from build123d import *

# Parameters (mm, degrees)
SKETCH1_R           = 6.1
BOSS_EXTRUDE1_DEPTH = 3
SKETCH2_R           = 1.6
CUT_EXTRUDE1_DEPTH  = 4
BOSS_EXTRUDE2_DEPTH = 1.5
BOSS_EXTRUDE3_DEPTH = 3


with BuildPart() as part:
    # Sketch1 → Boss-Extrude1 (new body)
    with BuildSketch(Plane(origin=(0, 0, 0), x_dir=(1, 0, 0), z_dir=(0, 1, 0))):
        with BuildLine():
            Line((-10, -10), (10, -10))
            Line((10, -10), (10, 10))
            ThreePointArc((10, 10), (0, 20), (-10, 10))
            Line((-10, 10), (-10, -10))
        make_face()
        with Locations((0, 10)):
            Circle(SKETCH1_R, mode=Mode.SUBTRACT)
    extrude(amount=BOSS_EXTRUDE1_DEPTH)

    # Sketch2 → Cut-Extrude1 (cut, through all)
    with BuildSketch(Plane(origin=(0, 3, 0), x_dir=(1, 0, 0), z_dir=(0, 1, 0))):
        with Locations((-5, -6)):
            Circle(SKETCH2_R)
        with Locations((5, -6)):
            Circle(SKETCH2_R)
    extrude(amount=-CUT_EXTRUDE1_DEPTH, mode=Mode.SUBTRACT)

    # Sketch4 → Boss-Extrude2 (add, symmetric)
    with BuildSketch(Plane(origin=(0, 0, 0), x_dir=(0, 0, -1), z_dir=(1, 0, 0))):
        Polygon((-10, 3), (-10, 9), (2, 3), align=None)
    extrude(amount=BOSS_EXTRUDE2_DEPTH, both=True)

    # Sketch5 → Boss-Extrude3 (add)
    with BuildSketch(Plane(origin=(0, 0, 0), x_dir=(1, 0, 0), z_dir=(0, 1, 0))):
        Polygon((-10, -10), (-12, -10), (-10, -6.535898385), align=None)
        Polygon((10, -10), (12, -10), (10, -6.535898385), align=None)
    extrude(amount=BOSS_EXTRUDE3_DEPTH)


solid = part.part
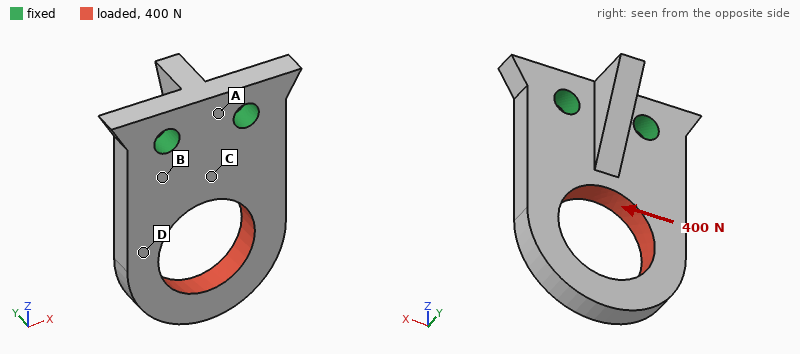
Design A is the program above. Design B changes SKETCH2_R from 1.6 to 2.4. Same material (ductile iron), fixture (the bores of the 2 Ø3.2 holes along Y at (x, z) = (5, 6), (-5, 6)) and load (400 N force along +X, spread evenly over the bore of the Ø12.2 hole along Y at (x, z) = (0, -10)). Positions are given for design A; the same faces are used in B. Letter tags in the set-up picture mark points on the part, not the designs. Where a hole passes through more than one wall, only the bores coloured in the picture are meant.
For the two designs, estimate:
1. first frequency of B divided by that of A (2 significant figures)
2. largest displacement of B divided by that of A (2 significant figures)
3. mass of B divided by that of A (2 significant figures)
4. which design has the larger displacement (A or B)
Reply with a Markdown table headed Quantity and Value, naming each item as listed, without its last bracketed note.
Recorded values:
| Quantity | Value |
|---|---|
| first frequency of B divided by that of A | 1.1 |
| largest displacement of B divided by that of A | 0.91 |
| mass of B divided by that of A | 0.96 |
| which design has the larger displacement | A |
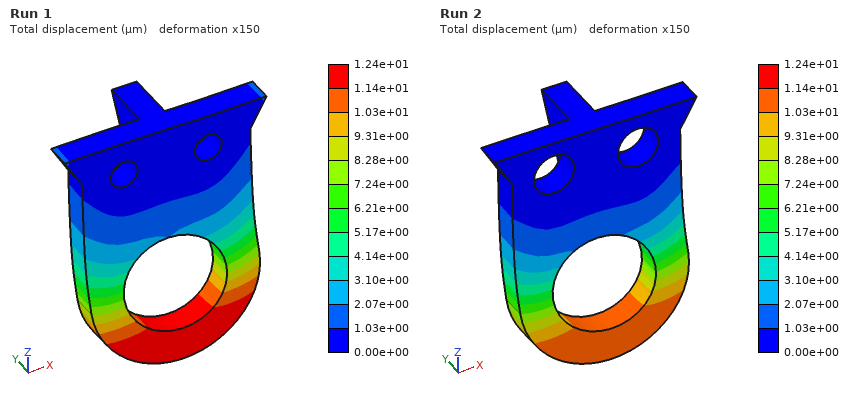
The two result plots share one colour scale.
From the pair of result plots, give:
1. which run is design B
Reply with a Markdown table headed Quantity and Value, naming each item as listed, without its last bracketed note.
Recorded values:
| Quantity | Value |
|---|---|
| which run is design B | Run 2 |
